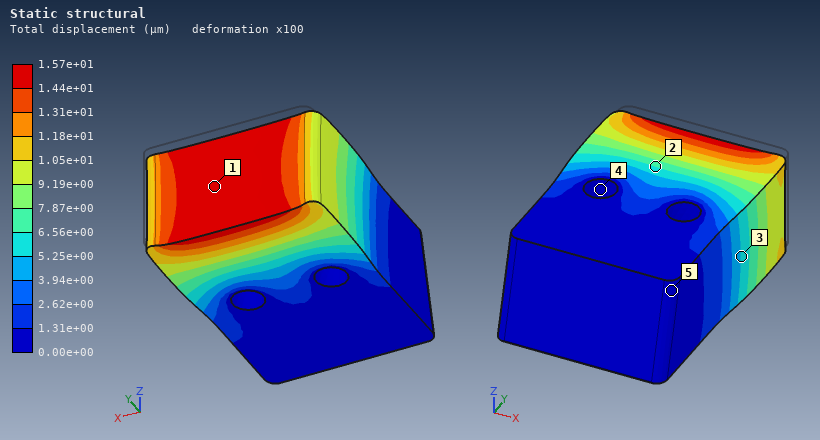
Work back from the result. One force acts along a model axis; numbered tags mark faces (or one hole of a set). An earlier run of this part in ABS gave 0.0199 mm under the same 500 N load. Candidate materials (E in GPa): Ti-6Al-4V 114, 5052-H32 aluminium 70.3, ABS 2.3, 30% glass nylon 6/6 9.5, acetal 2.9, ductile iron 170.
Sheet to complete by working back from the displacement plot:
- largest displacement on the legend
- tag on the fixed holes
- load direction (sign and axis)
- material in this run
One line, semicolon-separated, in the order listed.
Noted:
1.57e+01 µm; 4; -Y; acetal
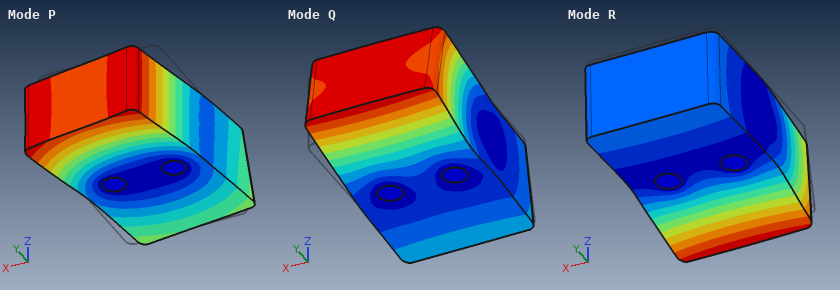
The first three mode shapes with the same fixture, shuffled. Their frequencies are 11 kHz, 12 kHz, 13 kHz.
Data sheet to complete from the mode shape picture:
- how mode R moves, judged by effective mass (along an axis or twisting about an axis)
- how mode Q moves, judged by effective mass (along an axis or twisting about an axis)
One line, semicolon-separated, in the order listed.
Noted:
along Z; along Z
